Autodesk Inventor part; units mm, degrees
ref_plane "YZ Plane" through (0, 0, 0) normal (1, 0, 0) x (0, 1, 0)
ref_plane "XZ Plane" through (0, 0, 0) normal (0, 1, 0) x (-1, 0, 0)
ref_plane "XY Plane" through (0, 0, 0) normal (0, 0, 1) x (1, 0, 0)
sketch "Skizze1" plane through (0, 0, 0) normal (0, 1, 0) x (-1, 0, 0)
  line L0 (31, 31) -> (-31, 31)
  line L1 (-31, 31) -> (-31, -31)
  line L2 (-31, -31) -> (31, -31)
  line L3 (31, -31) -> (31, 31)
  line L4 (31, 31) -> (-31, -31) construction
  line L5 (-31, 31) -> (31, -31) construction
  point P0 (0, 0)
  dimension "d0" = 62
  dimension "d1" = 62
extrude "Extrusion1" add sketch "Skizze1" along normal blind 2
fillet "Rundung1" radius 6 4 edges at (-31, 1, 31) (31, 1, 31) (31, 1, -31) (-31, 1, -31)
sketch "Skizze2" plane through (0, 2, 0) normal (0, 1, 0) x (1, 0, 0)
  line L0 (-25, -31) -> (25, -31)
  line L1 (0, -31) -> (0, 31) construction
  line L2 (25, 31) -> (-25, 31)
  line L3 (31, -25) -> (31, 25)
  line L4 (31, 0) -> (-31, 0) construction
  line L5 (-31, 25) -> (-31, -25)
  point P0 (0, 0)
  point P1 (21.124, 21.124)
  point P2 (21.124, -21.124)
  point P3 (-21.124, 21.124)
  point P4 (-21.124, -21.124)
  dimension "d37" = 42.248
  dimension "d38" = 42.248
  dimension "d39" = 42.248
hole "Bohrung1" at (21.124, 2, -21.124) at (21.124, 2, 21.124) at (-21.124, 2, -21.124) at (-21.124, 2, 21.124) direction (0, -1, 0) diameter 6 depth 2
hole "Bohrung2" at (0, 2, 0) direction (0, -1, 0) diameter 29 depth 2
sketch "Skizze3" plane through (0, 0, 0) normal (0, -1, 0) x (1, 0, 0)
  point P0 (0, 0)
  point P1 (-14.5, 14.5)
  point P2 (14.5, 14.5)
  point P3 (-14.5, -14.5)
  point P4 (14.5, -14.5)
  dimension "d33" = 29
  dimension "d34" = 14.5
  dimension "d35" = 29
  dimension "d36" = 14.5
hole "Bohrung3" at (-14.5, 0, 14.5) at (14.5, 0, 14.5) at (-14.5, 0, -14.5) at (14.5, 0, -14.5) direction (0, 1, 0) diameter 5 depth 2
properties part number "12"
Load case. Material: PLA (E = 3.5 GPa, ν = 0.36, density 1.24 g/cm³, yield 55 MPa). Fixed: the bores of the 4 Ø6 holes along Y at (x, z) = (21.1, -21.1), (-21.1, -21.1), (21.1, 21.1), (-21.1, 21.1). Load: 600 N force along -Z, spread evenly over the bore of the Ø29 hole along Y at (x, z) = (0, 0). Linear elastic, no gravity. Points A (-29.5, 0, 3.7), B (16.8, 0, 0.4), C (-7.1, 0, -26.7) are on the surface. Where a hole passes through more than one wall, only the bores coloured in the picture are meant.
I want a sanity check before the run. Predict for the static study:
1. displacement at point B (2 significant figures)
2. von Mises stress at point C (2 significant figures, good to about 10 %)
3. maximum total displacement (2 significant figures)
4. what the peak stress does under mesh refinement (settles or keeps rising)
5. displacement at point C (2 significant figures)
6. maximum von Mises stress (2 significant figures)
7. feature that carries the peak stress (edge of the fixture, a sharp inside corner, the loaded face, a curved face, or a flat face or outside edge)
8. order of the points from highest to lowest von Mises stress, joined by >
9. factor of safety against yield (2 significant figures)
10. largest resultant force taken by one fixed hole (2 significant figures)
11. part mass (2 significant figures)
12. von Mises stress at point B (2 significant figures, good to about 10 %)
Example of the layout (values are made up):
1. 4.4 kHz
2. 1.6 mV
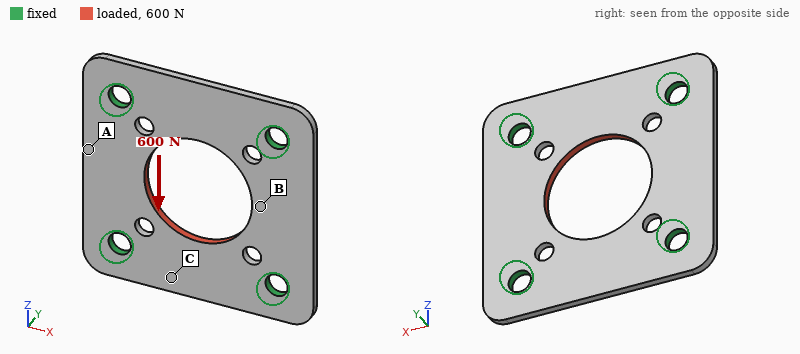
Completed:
1. 22 µm
2. 2.8 MPa
3. 47 µm
4. settles
5. 34 µm
6. 14 MPa
7. a curved face
8. B > C > A
9. 3.9
10. 150 N
11. 7.3 g
12. 5.4 MPa
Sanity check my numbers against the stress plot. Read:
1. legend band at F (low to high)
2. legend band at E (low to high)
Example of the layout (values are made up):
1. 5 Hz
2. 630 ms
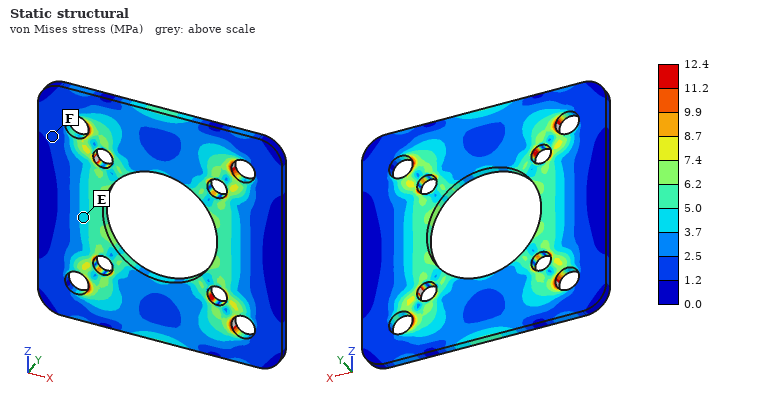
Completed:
1. 1.2 to 2.5 MPa
2. 3.7 to 5.0 MPa
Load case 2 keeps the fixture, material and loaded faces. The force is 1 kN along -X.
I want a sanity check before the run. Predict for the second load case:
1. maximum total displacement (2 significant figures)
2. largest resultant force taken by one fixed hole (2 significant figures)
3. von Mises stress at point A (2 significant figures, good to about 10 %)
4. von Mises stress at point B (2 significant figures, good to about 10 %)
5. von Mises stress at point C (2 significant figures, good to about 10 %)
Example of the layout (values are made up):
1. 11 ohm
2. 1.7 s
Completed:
1. 78 µm
2. 260 N
3. 6.5 MPa
4. 4.8 MPa
5. 2.0 MPa
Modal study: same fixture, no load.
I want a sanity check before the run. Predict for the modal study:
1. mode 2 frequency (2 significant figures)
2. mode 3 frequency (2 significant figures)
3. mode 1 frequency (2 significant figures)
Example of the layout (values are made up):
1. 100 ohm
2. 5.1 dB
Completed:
1. 2300 Hz
2. 2300 Hz
3. 2200 Hz
